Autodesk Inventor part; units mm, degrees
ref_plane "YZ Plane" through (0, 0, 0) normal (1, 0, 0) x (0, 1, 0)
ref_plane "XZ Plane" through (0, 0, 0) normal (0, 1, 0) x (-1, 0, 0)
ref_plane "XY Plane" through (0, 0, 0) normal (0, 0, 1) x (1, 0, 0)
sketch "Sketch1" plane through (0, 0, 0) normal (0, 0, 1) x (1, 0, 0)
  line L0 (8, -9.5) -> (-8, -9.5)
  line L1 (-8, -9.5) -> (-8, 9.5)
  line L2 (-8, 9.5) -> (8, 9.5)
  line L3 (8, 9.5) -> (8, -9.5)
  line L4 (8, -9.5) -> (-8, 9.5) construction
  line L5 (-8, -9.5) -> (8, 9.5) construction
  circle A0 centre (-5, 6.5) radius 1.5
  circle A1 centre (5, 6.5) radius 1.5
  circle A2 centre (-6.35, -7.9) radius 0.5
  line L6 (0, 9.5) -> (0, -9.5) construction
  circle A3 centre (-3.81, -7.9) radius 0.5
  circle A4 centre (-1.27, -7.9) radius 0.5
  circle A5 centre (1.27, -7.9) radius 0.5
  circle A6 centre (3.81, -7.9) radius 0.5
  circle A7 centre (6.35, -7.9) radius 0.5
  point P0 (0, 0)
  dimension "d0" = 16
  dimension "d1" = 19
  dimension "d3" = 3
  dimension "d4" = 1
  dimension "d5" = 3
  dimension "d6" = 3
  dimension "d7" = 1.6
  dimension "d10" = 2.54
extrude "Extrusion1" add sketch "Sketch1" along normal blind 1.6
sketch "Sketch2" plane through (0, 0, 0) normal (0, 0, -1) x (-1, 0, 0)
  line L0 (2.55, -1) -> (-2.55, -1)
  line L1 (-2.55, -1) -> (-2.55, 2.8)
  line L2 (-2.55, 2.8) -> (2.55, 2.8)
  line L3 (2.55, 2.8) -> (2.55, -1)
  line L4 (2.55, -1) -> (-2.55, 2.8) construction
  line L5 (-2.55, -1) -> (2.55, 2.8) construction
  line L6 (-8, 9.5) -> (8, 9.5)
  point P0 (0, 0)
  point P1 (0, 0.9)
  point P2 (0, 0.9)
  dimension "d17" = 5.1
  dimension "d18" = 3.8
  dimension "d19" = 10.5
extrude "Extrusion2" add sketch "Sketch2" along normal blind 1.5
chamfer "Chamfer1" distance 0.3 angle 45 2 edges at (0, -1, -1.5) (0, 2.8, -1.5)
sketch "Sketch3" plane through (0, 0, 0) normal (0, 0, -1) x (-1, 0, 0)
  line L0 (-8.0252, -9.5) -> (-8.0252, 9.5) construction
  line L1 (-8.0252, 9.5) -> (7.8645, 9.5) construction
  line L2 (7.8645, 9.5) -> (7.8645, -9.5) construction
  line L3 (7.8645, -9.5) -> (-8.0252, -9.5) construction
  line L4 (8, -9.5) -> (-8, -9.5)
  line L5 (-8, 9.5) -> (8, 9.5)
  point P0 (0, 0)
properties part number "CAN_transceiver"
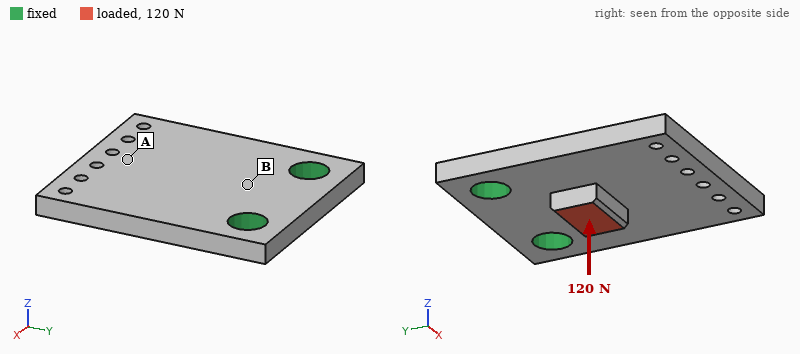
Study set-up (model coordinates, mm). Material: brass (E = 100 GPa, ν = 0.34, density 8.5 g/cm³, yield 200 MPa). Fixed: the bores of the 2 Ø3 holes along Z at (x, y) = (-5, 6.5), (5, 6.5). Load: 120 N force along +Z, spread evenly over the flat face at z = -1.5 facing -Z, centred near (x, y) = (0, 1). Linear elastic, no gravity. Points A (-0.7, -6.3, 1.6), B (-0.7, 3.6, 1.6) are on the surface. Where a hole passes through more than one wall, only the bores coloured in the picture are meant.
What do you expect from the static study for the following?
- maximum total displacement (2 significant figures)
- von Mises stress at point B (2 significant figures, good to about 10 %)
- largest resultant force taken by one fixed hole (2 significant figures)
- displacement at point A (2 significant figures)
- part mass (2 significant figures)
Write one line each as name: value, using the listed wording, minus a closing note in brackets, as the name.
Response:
maximum total displacement: 37 µm
von Mises stress at point B: 33 MPa
largest resultant force taken by one fixed hole: 60 N
displacement at point A: 29 µm
part mass: 4.1 g
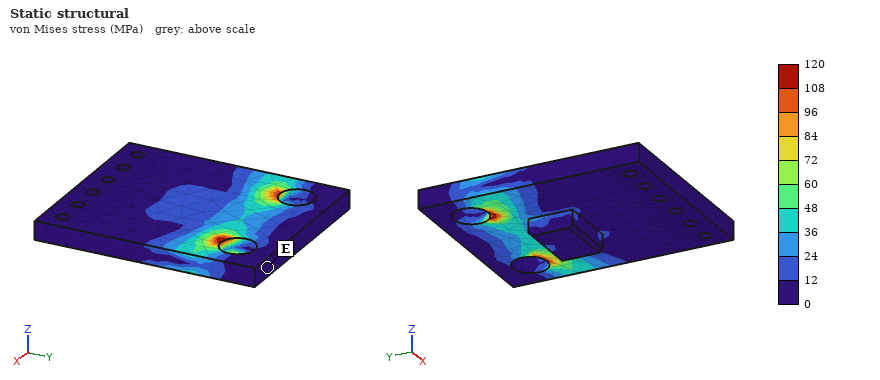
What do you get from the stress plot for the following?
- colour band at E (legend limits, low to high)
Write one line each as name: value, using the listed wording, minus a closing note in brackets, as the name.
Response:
colour band at E: 0 to 12 MPa
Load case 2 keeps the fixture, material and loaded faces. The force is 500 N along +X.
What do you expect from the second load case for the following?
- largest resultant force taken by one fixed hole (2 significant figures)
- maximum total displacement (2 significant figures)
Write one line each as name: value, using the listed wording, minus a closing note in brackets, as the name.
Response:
largest resultant force taken by one fixed hole: 350 N
maximum total displacement: 20 µm
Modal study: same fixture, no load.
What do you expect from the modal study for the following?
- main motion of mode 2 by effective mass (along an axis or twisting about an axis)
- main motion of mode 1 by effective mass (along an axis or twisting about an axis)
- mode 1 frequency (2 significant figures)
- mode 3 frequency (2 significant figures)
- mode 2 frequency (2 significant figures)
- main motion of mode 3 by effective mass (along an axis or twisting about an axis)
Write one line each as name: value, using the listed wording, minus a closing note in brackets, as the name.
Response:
main motion of mode 2 by effective mass: twisting about Y
main motion of mode 1 by effective mass: along Z
mode 1 frequency: 4200 Hz
mode 3 frequency: 23 kHz
mode 2 frequency: 9700 Hz
main motion of mode 3 by effective mass: along Z
